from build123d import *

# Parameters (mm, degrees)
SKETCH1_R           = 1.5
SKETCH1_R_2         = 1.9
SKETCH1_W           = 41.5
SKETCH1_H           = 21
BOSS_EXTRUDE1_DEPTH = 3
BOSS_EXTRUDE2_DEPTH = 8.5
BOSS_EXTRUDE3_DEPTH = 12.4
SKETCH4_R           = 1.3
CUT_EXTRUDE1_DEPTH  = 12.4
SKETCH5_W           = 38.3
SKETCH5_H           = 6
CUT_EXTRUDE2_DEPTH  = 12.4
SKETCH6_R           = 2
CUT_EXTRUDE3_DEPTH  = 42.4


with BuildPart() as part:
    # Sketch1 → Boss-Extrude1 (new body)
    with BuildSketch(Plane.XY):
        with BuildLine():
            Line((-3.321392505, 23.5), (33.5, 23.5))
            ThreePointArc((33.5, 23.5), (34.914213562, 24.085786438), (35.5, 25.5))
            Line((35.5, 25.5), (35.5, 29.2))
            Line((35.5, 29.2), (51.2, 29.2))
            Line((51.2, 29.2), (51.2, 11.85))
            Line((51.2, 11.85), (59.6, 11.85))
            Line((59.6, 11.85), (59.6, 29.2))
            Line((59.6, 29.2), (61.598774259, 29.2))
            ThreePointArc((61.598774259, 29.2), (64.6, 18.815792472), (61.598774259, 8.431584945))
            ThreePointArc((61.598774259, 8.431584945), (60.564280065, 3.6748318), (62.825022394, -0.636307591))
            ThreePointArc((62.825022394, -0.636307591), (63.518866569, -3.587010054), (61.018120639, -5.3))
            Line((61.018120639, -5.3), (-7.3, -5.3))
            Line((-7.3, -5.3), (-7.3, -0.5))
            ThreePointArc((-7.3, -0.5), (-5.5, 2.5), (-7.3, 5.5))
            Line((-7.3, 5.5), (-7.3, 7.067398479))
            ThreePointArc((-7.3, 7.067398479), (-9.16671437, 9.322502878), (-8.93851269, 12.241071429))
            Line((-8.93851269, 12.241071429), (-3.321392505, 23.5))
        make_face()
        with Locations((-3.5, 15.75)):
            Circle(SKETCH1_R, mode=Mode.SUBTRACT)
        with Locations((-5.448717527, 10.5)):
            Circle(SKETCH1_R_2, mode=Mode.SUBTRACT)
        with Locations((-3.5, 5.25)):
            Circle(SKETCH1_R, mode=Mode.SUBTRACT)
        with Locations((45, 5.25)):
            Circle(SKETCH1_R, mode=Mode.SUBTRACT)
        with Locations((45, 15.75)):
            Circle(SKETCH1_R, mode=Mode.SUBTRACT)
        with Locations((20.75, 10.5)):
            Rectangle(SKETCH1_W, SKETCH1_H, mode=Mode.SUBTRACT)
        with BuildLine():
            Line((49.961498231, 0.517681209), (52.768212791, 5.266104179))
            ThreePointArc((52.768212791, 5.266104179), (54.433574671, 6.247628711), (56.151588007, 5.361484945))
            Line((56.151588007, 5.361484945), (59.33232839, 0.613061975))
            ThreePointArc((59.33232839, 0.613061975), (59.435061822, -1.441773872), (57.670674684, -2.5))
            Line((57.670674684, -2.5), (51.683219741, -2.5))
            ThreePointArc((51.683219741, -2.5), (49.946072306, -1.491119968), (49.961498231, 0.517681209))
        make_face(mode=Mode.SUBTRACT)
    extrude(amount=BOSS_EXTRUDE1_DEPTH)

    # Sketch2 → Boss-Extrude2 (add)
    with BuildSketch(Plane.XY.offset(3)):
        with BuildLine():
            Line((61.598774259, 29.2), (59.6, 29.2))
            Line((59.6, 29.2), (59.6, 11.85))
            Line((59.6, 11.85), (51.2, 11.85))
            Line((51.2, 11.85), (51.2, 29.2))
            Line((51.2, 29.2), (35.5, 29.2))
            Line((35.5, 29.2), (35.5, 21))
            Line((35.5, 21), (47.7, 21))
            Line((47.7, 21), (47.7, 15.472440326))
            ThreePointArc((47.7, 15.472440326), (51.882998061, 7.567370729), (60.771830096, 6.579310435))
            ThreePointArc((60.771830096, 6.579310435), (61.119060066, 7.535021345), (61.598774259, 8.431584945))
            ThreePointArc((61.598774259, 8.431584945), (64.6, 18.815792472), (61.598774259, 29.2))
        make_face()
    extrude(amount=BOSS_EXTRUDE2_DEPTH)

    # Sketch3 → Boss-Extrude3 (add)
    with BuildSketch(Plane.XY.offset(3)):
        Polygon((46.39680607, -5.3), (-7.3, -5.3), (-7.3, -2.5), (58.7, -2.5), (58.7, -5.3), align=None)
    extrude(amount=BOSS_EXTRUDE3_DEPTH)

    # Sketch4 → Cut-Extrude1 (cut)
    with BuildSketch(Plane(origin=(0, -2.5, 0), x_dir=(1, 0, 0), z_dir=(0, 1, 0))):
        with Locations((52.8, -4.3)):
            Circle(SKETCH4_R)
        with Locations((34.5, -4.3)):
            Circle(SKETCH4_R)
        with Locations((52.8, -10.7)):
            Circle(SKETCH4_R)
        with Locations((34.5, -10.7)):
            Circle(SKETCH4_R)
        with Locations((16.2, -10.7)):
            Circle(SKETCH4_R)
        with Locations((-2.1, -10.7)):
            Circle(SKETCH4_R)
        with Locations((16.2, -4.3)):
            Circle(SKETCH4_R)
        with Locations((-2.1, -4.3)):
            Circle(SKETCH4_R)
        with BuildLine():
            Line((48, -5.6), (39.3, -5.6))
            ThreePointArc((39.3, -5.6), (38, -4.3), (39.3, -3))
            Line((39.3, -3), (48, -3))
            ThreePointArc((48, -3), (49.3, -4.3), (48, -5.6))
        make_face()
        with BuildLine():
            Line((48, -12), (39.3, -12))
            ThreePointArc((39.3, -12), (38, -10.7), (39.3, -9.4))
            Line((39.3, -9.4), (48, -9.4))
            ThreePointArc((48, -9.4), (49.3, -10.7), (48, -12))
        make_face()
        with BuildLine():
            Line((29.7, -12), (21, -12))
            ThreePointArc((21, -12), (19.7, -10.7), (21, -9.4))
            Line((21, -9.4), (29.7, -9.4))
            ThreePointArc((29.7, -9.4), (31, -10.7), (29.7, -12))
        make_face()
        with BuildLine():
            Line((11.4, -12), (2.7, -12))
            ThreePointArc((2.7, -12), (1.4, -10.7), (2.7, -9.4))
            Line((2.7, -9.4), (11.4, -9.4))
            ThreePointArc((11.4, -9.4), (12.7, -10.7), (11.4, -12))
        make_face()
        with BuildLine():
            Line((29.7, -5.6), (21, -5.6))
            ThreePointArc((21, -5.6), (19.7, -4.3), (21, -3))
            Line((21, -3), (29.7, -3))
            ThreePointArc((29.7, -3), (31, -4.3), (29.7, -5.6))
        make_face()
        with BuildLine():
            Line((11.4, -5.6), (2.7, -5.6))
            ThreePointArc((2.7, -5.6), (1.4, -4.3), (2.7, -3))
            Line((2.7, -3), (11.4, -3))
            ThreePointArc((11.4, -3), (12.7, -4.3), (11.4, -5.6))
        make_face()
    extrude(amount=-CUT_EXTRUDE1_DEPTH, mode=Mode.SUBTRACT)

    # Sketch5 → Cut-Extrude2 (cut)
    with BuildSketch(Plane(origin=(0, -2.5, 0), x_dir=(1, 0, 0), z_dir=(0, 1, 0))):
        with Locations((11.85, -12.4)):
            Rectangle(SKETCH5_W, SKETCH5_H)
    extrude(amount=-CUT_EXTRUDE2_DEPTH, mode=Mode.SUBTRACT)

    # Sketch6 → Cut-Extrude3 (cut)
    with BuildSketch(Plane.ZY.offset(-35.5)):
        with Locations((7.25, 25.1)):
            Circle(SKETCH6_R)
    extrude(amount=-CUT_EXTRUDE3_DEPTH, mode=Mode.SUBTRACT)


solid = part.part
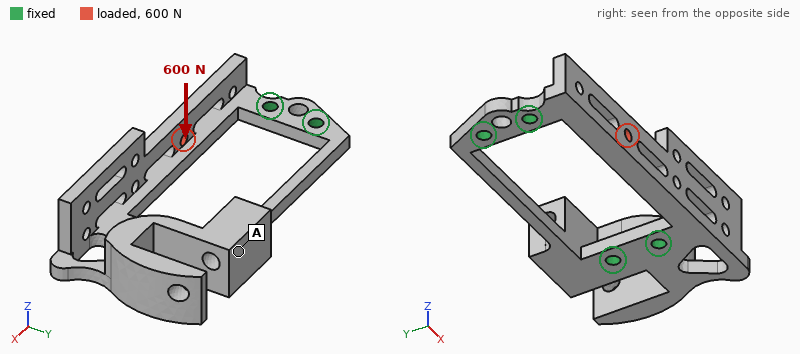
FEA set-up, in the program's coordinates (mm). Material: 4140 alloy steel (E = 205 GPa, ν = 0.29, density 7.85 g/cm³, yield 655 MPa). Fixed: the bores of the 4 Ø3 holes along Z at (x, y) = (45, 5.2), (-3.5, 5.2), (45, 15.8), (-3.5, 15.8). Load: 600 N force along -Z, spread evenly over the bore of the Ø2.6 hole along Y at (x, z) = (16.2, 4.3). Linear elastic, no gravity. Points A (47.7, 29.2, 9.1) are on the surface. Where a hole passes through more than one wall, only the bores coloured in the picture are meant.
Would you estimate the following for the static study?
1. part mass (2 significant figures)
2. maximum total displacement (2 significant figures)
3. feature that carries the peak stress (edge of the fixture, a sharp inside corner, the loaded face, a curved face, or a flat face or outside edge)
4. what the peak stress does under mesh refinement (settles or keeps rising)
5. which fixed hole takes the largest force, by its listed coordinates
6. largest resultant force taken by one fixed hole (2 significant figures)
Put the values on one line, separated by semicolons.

52 g; 72 µm; edge of the fixture; keeps rising; (-3.5, 5.2); 380 N
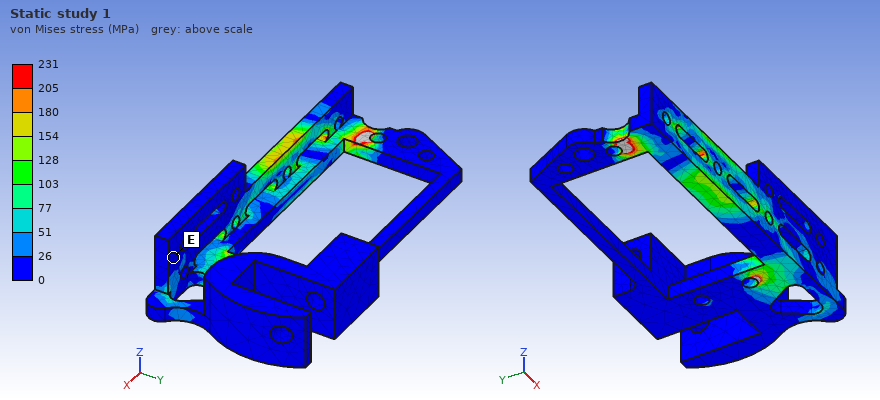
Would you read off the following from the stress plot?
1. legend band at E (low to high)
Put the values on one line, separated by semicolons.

0 to 26 MPa
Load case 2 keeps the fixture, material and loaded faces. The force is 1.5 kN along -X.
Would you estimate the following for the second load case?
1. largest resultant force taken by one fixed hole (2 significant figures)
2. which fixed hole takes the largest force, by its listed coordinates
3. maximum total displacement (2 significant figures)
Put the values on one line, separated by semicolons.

1.2 kN; (45, 5.2); 16 µm
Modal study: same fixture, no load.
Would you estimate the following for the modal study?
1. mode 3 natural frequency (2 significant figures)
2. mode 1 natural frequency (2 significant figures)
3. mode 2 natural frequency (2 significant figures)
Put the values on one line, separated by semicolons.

5800 Hz; 3900 Hz; 4300 Hz
